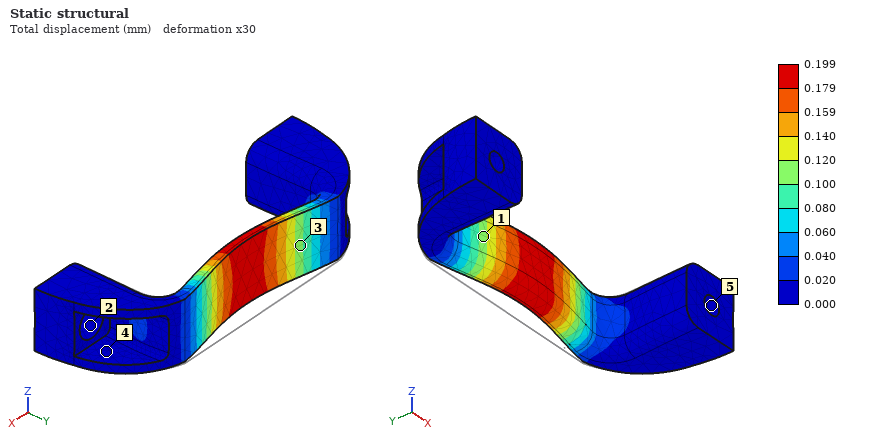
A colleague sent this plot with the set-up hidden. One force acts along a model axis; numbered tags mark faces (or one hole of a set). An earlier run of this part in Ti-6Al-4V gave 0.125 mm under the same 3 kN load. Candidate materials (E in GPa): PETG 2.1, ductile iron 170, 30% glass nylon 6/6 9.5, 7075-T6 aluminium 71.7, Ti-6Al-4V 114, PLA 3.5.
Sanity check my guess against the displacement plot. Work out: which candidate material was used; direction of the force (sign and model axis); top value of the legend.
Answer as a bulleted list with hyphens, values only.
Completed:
- 7075-T6 aluminium
- -Y
- 0.199 mm
